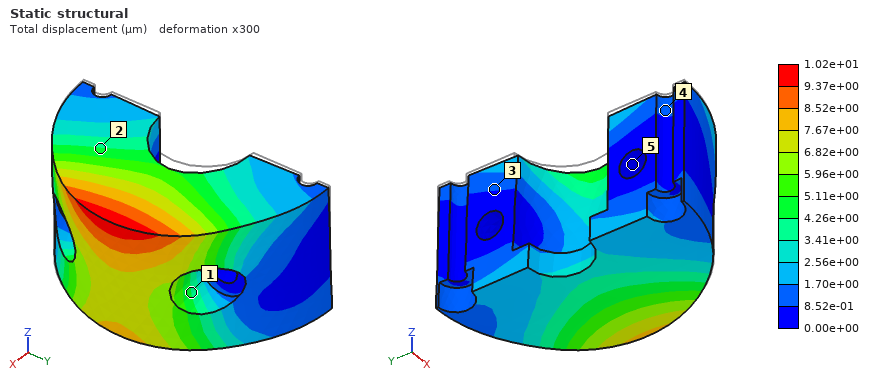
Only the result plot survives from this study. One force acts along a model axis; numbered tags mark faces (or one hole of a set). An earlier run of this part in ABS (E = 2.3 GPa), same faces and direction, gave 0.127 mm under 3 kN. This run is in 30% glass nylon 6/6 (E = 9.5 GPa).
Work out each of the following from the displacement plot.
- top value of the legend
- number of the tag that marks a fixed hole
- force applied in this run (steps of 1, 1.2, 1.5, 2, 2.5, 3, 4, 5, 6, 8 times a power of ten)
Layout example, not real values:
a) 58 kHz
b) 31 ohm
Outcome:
a) 1.02e+01 µm
b) 5
c) 1 kN
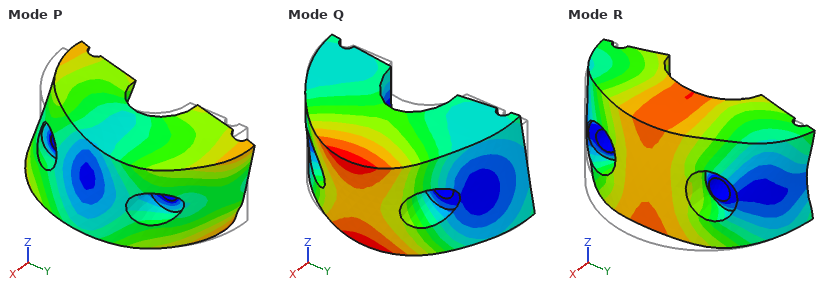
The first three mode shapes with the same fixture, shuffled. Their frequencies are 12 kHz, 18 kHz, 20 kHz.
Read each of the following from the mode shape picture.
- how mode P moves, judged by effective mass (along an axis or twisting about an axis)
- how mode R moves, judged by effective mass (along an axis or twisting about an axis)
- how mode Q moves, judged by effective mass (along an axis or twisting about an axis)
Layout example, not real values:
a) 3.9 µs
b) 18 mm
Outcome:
a) twisting about X
b) along X
c) along Z
